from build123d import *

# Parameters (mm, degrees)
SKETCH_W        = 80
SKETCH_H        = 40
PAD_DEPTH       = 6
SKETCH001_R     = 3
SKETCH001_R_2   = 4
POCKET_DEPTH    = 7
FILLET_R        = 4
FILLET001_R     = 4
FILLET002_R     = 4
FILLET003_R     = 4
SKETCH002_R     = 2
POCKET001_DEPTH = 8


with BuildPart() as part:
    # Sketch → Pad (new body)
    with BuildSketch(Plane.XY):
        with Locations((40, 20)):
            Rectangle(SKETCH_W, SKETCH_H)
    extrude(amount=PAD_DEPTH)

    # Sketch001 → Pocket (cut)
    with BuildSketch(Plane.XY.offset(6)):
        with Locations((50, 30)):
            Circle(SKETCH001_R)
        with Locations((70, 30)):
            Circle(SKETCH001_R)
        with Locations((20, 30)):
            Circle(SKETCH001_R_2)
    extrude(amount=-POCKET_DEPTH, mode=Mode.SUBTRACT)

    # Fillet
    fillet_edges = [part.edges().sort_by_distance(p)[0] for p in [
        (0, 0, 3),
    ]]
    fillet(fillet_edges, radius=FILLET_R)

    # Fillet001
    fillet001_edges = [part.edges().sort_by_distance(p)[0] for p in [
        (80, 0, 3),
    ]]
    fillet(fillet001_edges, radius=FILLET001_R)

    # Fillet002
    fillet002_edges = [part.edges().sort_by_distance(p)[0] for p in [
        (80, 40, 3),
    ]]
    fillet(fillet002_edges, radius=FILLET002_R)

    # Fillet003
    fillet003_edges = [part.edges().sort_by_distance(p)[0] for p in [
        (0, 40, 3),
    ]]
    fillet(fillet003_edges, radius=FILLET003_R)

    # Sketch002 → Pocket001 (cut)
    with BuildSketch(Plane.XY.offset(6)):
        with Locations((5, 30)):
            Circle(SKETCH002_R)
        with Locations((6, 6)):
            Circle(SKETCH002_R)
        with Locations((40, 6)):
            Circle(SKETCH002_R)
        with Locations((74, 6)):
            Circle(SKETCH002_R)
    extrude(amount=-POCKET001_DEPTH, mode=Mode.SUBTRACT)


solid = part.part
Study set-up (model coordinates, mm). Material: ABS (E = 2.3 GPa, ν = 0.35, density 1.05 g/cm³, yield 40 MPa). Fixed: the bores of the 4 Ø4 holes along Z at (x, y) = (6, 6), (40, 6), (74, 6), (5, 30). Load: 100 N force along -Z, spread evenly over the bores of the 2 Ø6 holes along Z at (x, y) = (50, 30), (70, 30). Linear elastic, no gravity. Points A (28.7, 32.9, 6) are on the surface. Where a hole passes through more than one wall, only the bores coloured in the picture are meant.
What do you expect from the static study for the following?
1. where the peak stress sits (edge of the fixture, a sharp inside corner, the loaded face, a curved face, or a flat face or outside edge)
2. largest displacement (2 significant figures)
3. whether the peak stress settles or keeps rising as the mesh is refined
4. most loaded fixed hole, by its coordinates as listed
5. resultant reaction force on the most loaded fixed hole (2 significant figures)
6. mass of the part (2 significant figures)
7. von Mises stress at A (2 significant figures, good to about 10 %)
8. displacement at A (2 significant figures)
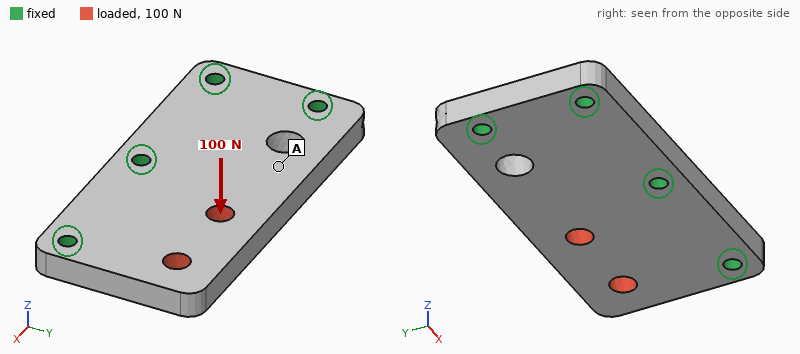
edge of the fixture
0.44 mm
keeps rising
(74, 6)
57 N
19 g
2.3 MPa
0.11 mm
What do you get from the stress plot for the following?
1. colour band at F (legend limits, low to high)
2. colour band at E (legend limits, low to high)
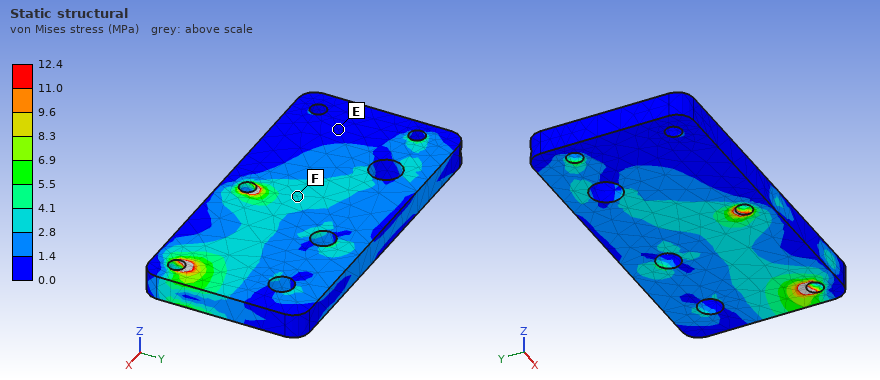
2.8 to 4.1 MPa
0.0 to 1.4 MPa
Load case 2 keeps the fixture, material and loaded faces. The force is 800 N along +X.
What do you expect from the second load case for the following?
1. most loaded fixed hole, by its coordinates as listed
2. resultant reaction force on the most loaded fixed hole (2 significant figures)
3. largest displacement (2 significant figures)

(74, 6)
350 N
0.10 mm
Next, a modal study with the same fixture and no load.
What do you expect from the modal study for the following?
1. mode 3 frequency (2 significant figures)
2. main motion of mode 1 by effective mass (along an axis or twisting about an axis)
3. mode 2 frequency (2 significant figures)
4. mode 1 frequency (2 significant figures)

4700 Hz
along Z
2600 Hz
1300 Hz
